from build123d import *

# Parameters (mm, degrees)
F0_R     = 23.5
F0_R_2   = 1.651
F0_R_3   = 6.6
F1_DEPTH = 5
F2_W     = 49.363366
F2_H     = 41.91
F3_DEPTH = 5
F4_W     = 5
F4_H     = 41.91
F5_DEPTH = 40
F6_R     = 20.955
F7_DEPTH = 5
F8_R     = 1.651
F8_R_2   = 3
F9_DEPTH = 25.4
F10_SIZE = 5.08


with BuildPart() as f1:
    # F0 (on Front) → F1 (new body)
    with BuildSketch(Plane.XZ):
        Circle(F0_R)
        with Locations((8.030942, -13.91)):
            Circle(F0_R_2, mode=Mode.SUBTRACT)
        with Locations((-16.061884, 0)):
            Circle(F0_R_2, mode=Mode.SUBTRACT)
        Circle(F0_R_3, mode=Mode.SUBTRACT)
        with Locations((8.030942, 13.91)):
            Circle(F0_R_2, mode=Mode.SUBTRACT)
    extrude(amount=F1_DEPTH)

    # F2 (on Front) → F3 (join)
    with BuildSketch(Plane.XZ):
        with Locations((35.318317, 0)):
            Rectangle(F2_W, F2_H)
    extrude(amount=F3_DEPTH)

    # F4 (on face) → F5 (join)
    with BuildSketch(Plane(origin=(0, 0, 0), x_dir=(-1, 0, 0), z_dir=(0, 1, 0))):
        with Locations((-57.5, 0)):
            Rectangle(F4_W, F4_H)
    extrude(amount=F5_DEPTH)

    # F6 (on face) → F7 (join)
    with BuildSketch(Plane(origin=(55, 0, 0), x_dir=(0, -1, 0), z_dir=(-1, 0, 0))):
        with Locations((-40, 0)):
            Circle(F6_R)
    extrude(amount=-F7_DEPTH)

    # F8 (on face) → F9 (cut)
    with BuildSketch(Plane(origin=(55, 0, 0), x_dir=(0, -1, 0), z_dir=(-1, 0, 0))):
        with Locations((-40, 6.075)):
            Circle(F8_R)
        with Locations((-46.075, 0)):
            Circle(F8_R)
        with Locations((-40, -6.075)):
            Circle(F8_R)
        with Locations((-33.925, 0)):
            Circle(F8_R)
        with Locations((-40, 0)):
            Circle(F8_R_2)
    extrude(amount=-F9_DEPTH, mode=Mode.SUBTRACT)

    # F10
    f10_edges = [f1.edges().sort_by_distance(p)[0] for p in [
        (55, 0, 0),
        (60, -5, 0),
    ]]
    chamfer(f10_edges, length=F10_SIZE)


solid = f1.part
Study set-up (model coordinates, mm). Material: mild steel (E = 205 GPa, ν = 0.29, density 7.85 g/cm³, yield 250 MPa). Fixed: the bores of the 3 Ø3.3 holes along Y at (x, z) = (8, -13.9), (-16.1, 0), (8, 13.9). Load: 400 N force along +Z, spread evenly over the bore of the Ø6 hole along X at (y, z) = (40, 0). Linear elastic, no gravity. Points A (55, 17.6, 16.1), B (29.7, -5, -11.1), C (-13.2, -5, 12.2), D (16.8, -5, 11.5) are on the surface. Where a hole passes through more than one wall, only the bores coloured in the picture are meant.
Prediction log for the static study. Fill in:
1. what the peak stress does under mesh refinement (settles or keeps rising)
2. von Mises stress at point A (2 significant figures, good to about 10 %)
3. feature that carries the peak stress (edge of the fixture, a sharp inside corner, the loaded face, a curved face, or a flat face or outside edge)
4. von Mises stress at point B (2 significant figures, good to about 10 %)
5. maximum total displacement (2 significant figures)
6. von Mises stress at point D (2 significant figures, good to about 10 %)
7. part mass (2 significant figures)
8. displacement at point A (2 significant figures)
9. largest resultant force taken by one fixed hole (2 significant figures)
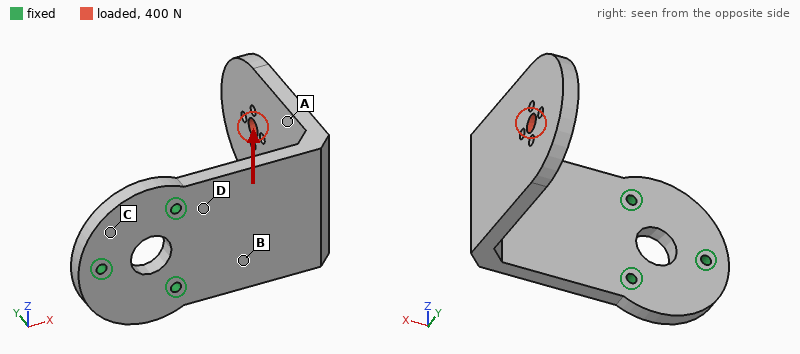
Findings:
keeps rising
16 MPa
edge of the fixture
70 MPa
0.27 mm
60 MPa
220 g
0.11 mm
860 N
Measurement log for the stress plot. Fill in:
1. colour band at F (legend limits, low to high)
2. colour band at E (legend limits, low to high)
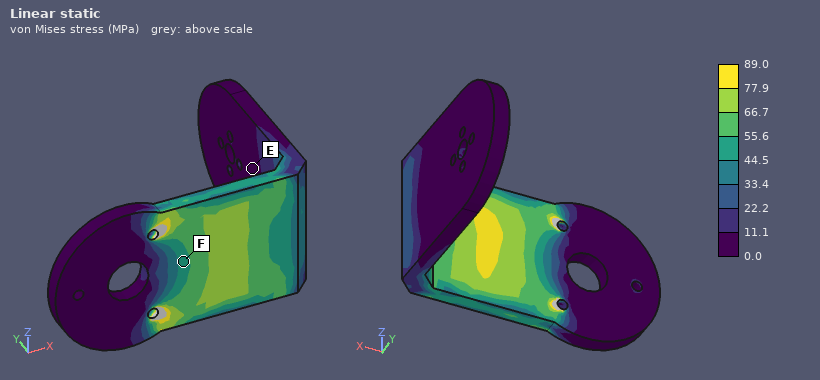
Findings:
44.5 to 55.6 MPa
0.0 to 11.1 MPa
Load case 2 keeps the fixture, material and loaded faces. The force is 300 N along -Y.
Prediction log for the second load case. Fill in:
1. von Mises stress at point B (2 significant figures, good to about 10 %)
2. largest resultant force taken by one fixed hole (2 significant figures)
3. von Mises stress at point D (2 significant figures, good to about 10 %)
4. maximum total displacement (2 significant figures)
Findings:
45 MPa
210 N
67 MPa
0.31 mm
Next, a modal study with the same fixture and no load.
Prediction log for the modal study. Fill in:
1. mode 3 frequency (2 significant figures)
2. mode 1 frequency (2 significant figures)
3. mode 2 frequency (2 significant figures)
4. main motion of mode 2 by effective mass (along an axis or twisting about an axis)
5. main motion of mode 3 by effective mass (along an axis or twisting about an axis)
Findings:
1400 Hz
480 Hz
900 Hz
along Z
along Y
